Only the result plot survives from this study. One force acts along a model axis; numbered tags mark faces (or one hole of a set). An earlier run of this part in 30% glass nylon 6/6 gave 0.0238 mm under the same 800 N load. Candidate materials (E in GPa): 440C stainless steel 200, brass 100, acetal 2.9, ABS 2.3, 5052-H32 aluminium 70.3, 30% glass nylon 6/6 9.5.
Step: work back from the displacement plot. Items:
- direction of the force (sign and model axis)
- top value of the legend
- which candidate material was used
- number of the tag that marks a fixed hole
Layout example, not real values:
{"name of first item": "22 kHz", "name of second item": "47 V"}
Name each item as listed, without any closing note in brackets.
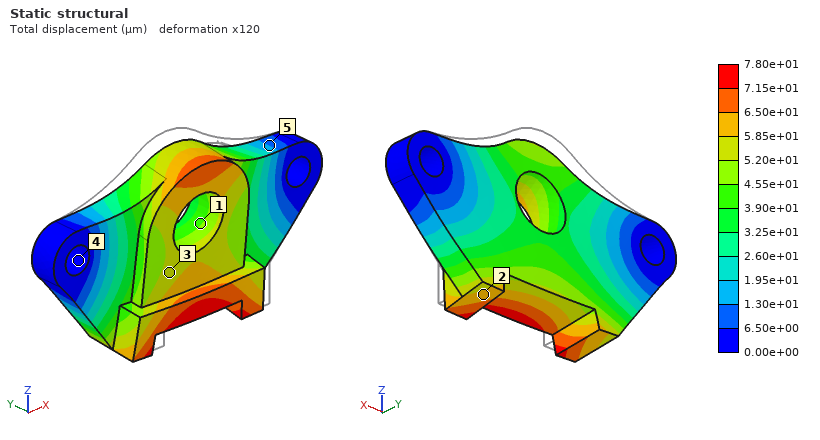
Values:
{"direction of the force": "-Z", "top value of the legend": "7.80e+01 µm", "which candidate material was used": "acetal", "number of the tag that marks a fixed hole": "4"}
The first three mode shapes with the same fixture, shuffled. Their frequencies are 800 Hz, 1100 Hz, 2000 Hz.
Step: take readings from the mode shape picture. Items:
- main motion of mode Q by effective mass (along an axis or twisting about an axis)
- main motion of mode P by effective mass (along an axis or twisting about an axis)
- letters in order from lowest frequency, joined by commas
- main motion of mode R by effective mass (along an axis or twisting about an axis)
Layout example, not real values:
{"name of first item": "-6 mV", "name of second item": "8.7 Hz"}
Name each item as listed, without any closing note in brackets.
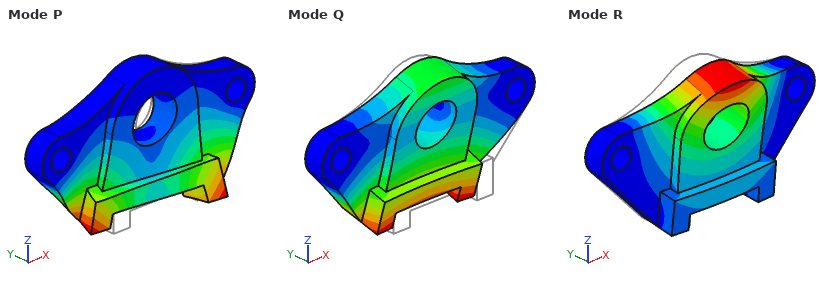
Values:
{"main motion of mode Q by effective mass": "along Y", "main motion of mode P by effective mass": "twisting about Z", "letters in order from lowest frequency, joined by commas": "Q, R, P", "main motion of mode R by effective mass": "along Y"}
